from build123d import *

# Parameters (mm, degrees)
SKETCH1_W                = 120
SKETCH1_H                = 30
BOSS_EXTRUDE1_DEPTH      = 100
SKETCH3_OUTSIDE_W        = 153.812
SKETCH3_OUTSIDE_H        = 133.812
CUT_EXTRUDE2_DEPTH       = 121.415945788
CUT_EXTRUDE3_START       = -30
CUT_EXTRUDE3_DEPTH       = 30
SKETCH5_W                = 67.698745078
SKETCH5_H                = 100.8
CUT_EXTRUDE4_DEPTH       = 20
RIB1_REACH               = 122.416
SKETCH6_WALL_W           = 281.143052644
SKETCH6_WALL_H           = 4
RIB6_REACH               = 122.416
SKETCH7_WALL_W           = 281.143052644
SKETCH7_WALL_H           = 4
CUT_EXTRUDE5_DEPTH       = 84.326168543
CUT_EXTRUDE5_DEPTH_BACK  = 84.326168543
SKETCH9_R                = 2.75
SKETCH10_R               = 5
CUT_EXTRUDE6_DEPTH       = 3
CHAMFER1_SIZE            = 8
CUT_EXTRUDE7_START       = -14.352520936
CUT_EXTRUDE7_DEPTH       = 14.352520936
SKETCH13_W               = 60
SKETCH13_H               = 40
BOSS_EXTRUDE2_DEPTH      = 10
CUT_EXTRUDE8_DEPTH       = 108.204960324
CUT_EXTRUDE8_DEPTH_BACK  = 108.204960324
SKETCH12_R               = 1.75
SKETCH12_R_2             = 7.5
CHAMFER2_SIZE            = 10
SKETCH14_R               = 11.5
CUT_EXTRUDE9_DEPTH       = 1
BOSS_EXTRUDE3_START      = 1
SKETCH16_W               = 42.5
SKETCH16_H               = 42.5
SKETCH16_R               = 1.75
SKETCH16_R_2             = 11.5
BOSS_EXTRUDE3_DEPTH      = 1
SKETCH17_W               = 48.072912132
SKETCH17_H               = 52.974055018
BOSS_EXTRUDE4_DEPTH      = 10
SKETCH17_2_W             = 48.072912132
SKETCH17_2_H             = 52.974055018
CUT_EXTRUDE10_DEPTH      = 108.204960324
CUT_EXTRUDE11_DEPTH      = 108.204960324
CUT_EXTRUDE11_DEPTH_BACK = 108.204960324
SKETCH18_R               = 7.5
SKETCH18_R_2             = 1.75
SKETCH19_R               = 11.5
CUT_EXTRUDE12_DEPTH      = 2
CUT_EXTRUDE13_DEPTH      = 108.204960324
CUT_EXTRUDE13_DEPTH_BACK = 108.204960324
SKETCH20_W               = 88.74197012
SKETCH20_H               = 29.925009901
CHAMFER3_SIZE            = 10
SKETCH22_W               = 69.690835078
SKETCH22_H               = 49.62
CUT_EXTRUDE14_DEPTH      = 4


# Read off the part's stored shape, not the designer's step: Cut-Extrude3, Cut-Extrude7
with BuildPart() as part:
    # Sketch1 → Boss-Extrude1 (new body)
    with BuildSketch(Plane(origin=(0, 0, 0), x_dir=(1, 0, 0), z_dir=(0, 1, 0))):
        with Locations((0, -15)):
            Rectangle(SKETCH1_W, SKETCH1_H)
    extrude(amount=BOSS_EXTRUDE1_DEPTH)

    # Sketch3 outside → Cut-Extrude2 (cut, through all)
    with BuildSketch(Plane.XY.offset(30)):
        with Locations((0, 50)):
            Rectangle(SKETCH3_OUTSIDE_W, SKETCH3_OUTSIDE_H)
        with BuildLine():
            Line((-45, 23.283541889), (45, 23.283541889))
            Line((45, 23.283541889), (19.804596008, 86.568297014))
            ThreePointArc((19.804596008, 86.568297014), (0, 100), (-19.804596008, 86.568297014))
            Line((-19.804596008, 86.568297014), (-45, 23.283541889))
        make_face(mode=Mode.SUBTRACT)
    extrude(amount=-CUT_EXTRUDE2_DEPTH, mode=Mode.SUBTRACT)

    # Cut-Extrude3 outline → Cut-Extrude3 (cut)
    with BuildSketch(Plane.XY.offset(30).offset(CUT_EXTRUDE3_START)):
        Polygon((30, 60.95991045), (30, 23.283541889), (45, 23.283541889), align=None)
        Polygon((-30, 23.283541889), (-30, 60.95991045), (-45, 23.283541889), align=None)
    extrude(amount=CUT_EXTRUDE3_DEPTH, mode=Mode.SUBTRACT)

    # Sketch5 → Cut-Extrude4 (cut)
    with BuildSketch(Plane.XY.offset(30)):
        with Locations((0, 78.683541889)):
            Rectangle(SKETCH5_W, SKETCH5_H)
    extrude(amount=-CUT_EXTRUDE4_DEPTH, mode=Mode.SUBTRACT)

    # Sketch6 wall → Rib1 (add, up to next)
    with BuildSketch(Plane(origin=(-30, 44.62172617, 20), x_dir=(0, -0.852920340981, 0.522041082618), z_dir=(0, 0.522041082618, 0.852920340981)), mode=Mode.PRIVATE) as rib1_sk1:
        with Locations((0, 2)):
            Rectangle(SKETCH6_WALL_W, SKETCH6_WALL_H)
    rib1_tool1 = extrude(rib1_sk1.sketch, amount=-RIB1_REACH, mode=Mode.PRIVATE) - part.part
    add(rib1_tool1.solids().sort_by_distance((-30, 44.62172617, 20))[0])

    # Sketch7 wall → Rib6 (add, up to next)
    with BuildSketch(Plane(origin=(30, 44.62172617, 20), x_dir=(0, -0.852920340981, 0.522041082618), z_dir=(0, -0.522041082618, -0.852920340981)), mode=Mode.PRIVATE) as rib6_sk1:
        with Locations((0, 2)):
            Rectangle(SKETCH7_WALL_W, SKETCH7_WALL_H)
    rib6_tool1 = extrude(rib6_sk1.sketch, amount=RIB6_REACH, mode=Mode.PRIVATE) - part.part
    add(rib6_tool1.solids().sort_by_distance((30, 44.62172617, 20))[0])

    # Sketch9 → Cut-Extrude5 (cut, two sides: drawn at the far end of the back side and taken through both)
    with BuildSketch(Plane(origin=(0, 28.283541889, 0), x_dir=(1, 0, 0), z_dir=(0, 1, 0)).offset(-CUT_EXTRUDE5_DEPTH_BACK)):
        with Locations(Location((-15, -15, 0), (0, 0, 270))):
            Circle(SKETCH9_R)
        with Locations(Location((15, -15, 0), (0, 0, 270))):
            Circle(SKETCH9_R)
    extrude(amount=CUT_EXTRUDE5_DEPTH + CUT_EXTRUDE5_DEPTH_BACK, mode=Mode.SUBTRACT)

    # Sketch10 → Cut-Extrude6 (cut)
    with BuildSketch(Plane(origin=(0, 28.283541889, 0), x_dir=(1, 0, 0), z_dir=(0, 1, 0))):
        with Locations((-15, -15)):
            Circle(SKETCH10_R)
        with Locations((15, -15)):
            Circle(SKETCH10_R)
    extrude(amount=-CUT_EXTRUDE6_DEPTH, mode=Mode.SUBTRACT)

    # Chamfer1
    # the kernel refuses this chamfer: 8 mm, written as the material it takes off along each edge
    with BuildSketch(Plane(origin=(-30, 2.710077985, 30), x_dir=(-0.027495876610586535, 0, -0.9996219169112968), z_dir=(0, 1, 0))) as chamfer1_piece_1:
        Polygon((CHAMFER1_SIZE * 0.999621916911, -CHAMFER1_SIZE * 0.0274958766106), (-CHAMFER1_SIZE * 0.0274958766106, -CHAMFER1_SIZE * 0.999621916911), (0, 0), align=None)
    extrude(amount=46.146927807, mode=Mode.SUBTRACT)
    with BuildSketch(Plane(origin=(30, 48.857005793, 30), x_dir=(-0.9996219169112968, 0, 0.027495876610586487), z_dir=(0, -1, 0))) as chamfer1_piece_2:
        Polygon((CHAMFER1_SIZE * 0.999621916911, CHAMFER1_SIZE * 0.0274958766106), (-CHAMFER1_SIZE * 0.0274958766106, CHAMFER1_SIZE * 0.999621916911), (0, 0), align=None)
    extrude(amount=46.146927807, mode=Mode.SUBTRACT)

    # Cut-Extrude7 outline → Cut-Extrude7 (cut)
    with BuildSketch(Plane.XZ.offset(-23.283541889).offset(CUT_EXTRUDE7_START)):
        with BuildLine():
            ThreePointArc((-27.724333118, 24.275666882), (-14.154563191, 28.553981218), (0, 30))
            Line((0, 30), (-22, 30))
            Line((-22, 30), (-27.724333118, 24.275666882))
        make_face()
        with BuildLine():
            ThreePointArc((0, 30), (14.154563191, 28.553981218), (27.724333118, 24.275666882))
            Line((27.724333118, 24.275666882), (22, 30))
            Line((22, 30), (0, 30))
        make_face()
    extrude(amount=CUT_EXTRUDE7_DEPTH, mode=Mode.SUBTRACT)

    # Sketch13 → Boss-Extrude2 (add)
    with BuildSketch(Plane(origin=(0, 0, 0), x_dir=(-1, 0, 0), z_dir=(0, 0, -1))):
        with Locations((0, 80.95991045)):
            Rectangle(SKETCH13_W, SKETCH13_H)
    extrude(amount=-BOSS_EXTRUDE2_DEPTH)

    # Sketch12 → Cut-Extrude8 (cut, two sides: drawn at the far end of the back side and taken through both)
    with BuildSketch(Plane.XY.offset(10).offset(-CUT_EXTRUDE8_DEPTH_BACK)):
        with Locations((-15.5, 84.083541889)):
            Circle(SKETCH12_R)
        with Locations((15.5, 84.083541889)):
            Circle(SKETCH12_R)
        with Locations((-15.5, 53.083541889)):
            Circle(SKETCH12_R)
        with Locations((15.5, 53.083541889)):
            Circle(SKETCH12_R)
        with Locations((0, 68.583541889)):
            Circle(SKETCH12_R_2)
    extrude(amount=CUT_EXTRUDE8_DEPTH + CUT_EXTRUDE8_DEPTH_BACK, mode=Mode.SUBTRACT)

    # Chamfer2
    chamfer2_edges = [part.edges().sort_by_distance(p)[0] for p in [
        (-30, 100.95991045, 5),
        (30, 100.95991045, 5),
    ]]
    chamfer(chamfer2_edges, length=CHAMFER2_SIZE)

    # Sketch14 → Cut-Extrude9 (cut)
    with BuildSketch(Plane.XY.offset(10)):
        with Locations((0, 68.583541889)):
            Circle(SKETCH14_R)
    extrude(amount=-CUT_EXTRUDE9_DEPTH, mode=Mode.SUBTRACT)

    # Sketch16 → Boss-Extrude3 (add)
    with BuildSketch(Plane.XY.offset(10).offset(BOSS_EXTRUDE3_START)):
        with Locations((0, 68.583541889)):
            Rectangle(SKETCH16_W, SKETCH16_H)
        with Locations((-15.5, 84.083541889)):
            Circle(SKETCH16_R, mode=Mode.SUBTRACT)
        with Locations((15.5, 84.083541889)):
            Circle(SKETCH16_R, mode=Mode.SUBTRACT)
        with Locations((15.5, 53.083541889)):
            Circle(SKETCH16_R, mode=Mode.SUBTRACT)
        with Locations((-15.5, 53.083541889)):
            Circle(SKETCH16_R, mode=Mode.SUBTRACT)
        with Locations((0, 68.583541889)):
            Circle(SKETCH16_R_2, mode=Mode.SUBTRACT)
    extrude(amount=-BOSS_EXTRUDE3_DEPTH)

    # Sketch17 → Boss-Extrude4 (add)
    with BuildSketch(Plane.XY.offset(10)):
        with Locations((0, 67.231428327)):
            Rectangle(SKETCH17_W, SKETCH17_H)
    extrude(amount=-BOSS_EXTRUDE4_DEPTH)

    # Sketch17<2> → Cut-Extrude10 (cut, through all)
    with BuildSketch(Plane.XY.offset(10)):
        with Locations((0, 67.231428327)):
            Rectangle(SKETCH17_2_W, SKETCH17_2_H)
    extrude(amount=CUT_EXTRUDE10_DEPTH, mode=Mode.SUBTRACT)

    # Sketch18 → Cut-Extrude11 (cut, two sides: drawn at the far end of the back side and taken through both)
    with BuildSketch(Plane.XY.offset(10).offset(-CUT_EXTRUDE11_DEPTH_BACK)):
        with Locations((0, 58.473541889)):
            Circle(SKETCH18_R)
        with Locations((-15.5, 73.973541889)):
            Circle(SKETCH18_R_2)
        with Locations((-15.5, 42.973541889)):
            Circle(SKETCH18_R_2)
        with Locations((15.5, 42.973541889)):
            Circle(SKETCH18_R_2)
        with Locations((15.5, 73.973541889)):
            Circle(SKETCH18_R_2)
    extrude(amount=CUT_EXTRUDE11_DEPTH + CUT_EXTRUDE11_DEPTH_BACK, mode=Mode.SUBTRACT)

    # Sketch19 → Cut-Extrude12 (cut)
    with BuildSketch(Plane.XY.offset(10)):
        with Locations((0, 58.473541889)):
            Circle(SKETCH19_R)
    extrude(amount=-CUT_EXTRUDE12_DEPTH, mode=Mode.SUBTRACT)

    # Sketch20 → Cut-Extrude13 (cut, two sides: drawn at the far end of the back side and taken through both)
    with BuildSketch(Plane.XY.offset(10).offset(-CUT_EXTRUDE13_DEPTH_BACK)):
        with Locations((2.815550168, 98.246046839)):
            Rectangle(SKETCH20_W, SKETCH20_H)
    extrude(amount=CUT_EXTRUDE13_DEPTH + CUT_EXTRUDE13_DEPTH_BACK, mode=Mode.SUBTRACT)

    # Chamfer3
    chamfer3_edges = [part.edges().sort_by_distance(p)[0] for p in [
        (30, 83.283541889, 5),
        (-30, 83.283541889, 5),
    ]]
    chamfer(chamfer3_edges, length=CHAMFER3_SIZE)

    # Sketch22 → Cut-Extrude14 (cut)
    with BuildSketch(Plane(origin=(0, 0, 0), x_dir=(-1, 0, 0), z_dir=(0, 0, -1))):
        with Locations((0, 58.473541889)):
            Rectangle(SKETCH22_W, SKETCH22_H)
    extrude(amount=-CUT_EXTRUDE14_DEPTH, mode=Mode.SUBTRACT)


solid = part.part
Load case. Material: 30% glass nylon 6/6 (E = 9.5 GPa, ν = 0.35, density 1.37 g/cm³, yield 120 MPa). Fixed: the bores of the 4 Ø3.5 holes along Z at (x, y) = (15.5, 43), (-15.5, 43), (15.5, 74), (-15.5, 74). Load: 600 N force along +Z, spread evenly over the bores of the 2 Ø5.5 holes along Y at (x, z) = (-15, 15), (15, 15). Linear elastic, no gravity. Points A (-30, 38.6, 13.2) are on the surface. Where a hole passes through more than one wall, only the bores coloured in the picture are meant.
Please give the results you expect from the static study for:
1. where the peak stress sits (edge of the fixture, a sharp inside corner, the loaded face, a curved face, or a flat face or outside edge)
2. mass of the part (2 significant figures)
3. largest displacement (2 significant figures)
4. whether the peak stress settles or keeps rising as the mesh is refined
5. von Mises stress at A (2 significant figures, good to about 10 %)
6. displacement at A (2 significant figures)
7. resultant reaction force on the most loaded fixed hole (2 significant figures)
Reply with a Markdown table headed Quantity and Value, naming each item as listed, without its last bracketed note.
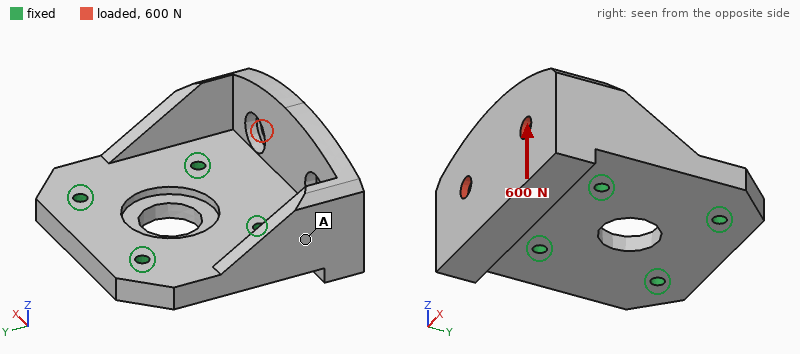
| Quantity | Value |
|---|---|
| where the peak stress sits | edge of the fixture |
| mass of the part | 40 g |
| largest displacement | 0.20 mm |
| whether the peak stress settles or keeps rising as the mesh is refined | keeps rising |
| von Mises stress at A | 4.1 MPa |
| displacement at A | 0.043 mm |
| resultant reaction force on the most loaded fixed hole | 400 N |
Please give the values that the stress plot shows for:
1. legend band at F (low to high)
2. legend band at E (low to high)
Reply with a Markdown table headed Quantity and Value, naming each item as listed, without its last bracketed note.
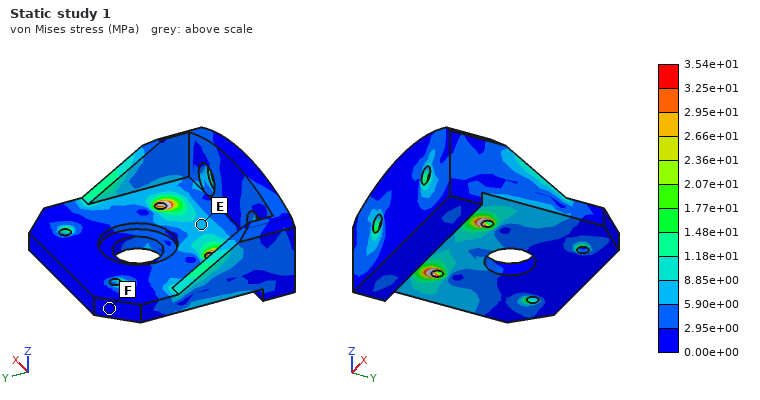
| Quantity | Value |
|---|---|
| legend band at F | 0.00e+00 to 2.95e+00 MPa |
| legend band at E | 5.90e+00 to 8.85e+00 MPa |
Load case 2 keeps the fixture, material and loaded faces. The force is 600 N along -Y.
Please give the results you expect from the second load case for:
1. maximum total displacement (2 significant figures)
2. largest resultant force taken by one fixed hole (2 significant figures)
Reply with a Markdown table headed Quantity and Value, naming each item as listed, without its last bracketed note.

| Quantity | Value |
|---|---|
| maximum total displacement | 0.13 mm |
| largest resultant force taken by one fixed hole | 260 N |
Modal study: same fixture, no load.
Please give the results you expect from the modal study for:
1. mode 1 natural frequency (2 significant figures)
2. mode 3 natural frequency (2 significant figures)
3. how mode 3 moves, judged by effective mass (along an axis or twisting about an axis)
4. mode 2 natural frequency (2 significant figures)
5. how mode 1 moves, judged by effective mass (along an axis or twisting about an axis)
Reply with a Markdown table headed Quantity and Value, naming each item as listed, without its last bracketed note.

| Quantity | Value |
|---|---|
| mode 1 natural frequency | 2800 Hz |
| mode 3 natural frequency | 5500 Hz |
| how mode 3 moves, judged by effective mass | along Z |
| mode 2 natural frequency | 3500 Hz |
| how mode 1 moves, judged by effective mass | along Z |
